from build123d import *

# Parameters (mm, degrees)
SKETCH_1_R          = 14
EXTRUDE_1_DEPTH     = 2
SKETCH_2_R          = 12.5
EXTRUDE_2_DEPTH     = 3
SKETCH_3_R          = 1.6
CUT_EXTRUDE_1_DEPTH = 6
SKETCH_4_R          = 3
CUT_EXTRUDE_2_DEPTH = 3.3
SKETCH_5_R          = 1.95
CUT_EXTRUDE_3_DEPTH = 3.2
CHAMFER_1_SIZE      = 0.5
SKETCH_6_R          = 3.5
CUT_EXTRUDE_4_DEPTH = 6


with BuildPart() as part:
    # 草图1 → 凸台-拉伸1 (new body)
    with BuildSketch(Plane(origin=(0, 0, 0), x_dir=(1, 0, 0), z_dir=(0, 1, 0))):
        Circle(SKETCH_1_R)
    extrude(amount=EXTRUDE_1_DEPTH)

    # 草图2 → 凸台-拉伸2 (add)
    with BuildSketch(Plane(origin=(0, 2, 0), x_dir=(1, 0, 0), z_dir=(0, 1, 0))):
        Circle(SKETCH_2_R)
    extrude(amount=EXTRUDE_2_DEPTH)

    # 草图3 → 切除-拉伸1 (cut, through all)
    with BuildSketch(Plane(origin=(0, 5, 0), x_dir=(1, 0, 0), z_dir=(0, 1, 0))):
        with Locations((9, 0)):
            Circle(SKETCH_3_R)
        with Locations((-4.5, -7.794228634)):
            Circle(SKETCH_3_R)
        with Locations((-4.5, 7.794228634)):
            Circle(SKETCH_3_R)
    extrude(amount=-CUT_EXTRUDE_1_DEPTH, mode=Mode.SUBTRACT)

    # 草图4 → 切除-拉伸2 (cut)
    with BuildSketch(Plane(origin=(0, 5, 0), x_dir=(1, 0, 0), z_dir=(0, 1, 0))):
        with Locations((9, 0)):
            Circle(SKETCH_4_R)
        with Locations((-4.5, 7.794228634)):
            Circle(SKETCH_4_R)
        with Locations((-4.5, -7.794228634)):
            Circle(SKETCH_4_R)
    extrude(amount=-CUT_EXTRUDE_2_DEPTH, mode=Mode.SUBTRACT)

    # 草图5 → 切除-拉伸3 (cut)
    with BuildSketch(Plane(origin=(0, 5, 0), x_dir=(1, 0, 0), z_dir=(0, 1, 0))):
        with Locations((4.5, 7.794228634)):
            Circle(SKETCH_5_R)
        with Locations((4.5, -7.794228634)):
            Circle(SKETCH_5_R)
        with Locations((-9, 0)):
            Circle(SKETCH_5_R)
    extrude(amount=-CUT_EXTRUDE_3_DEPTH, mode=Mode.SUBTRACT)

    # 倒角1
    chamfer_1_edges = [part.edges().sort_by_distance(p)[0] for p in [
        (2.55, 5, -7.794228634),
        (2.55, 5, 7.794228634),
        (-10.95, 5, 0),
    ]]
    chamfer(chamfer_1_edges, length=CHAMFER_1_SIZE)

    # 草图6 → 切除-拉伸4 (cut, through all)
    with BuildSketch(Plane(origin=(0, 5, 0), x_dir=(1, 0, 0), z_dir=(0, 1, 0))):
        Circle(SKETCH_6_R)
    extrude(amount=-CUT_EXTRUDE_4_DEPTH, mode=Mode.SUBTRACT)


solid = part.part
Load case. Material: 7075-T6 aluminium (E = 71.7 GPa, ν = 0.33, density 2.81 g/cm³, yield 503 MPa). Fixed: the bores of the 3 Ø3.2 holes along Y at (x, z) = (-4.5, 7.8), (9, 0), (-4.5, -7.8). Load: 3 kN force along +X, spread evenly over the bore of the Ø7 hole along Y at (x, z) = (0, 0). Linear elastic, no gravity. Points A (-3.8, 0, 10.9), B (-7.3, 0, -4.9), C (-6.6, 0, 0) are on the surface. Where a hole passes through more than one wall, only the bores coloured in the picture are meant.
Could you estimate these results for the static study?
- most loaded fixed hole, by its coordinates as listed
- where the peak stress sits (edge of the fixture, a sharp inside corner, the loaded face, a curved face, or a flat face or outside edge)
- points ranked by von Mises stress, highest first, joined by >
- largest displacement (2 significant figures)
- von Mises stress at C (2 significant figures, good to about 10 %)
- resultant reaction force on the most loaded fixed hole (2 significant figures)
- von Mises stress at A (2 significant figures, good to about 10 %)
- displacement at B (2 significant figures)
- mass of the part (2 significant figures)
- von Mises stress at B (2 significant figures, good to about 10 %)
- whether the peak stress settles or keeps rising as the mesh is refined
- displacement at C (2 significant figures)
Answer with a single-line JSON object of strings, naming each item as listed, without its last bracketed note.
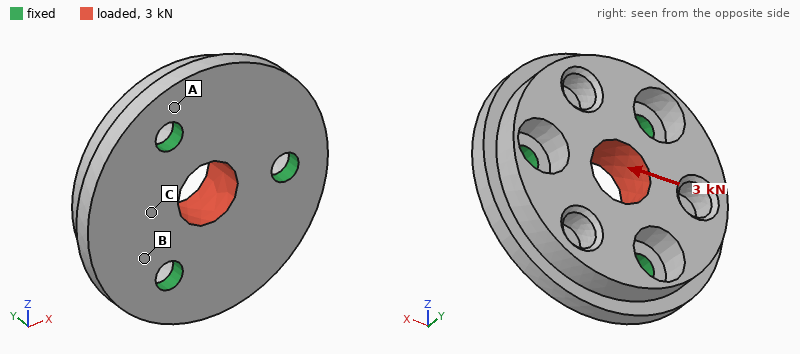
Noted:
{"most loaded fixed hole, by its coordinates as listed": "(9, 0)", "where the peak stress sits": "edge of the fixture", "points ranked by von Mises stress, highest first, joined by >": "B > C > A", "largest displacement": "13 µm", "von Mises stress at C": "31 MPa", "resultant reaction force on the most loaded fixed hole": "1.1 kN", "von Mises stress at A": "14 MPa", "displacement at B": "3.6 µm", "mass of the part": "5.8 g", "von Mises stress at B": "44 MPa", "whether the peak stress settles or keeps rising as the mesh is refined": "keeps rising", "displacement at C": "5.3 µm"}
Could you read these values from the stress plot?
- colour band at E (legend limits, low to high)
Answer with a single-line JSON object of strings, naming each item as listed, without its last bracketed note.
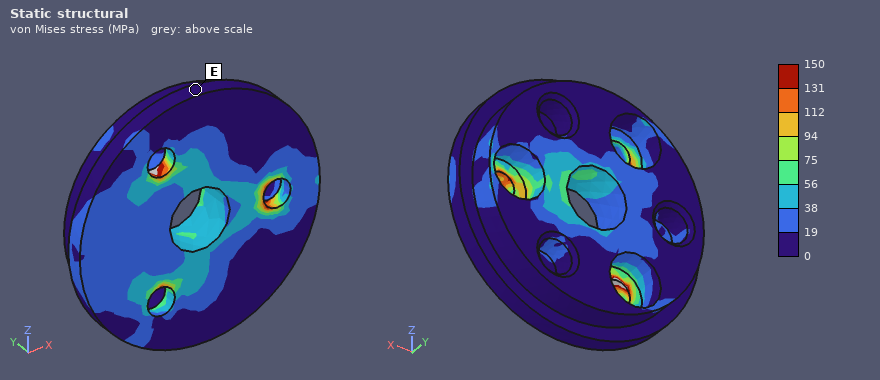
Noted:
{"colour band at E": "0 to 19 MPa"}
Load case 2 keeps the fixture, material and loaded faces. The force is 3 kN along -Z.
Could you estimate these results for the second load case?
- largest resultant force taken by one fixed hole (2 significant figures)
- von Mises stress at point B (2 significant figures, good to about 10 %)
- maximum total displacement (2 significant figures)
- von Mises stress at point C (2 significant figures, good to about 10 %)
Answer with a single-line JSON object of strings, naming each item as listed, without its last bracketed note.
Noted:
{"largest resultant force taken by one fixed hole": "1.1 kN", "von Mises stress at point B": "15 MPa", "maximum total displacement": "11 µm", "von Mises stress at point C": "13 MPa"}
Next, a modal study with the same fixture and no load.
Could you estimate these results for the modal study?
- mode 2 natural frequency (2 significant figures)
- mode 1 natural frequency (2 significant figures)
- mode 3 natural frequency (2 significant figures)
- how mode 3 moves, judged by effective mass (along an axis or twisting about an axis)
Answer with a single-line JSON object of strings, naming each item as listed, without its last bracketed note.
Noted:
{"mode 2 natural frequency": "26 kHz", "mode 1 natural frequency": "26 kHz", "mode 3 natural frequency": "34 kHz", "how mode 3 moves, judged by effective mass": "along Y"}
